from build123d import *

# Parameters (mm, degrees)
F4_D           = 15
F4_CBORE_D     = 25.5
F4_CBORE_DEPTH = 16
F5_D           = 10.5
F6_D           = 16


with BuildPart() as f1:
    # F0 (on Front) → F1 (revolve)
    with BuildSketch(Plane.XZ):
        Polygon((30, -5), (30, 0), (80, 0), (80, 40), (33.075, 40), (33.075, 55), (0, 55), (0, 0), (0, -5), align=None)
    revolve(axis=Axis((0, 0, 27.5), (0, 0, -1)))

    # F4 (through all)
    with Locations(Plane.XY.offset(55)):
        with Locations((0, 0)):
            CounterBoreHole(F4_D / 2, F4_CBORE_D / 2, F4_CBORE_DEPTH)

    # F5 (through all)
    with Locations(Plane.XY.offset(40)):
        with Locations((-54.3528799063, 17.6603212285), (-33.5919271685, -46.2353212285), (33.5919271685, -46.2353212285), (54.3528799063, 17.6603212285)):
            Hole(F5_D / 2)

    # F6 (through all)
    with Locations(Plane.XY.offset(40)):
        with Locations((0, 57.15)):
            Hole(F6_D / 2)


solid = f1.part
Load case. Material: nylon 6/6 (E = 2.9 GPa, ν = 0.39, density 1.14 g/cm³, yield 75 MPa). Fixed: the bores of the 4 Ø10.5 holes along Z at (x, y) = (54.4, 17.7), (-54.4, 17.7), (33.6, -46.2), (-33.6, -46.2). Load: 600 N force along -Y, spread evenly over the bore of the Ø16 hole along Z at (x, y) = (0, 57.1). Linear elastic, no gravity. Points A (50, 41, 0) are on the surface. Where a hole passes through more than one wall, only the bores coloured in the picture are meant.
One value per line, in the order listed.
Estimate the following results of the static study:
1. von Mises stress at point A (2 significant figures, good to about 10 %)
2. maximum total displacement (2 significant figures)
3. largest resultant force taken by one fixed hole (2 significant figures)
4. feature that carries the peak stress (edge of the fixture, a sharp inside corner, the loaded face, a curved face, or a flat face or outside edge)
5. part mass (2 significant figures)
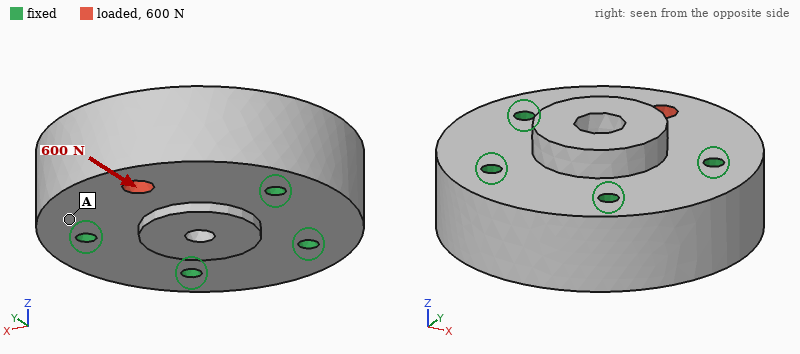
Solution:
0.091 MPa
7.3 µm
200 N
the loaded face
950 g
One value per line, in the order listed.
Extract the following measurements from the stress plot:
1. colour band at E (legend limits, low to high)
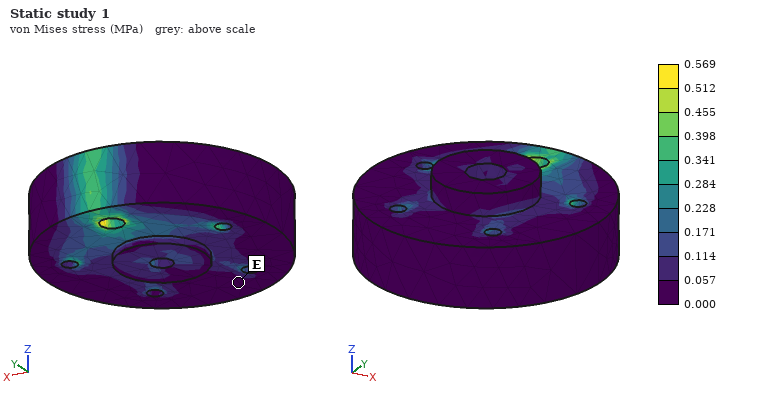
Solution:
0.000 to 0.057 MPa
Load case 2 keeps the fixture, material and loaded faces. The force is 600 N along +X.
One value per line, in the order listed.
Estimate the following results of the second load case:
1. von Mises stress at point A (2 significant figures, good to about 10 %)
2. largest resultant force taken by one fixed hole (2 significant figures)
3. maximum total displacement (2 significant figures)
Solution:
0.15 MPa
350 N
8.0 µm
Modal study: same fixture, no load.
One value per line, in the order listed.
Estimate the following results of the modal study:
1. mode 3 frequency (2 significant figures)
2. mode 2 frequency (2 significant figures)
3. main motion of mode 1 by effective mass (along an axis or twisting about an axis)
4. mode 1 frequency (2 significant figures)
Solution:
3800 Hz
3800 Hz
along Z
1900 Hz
